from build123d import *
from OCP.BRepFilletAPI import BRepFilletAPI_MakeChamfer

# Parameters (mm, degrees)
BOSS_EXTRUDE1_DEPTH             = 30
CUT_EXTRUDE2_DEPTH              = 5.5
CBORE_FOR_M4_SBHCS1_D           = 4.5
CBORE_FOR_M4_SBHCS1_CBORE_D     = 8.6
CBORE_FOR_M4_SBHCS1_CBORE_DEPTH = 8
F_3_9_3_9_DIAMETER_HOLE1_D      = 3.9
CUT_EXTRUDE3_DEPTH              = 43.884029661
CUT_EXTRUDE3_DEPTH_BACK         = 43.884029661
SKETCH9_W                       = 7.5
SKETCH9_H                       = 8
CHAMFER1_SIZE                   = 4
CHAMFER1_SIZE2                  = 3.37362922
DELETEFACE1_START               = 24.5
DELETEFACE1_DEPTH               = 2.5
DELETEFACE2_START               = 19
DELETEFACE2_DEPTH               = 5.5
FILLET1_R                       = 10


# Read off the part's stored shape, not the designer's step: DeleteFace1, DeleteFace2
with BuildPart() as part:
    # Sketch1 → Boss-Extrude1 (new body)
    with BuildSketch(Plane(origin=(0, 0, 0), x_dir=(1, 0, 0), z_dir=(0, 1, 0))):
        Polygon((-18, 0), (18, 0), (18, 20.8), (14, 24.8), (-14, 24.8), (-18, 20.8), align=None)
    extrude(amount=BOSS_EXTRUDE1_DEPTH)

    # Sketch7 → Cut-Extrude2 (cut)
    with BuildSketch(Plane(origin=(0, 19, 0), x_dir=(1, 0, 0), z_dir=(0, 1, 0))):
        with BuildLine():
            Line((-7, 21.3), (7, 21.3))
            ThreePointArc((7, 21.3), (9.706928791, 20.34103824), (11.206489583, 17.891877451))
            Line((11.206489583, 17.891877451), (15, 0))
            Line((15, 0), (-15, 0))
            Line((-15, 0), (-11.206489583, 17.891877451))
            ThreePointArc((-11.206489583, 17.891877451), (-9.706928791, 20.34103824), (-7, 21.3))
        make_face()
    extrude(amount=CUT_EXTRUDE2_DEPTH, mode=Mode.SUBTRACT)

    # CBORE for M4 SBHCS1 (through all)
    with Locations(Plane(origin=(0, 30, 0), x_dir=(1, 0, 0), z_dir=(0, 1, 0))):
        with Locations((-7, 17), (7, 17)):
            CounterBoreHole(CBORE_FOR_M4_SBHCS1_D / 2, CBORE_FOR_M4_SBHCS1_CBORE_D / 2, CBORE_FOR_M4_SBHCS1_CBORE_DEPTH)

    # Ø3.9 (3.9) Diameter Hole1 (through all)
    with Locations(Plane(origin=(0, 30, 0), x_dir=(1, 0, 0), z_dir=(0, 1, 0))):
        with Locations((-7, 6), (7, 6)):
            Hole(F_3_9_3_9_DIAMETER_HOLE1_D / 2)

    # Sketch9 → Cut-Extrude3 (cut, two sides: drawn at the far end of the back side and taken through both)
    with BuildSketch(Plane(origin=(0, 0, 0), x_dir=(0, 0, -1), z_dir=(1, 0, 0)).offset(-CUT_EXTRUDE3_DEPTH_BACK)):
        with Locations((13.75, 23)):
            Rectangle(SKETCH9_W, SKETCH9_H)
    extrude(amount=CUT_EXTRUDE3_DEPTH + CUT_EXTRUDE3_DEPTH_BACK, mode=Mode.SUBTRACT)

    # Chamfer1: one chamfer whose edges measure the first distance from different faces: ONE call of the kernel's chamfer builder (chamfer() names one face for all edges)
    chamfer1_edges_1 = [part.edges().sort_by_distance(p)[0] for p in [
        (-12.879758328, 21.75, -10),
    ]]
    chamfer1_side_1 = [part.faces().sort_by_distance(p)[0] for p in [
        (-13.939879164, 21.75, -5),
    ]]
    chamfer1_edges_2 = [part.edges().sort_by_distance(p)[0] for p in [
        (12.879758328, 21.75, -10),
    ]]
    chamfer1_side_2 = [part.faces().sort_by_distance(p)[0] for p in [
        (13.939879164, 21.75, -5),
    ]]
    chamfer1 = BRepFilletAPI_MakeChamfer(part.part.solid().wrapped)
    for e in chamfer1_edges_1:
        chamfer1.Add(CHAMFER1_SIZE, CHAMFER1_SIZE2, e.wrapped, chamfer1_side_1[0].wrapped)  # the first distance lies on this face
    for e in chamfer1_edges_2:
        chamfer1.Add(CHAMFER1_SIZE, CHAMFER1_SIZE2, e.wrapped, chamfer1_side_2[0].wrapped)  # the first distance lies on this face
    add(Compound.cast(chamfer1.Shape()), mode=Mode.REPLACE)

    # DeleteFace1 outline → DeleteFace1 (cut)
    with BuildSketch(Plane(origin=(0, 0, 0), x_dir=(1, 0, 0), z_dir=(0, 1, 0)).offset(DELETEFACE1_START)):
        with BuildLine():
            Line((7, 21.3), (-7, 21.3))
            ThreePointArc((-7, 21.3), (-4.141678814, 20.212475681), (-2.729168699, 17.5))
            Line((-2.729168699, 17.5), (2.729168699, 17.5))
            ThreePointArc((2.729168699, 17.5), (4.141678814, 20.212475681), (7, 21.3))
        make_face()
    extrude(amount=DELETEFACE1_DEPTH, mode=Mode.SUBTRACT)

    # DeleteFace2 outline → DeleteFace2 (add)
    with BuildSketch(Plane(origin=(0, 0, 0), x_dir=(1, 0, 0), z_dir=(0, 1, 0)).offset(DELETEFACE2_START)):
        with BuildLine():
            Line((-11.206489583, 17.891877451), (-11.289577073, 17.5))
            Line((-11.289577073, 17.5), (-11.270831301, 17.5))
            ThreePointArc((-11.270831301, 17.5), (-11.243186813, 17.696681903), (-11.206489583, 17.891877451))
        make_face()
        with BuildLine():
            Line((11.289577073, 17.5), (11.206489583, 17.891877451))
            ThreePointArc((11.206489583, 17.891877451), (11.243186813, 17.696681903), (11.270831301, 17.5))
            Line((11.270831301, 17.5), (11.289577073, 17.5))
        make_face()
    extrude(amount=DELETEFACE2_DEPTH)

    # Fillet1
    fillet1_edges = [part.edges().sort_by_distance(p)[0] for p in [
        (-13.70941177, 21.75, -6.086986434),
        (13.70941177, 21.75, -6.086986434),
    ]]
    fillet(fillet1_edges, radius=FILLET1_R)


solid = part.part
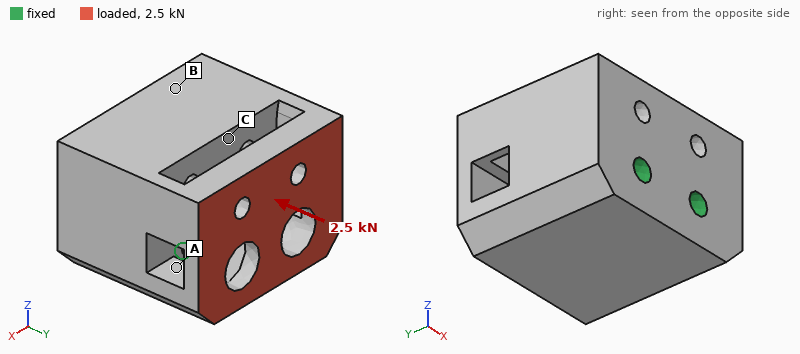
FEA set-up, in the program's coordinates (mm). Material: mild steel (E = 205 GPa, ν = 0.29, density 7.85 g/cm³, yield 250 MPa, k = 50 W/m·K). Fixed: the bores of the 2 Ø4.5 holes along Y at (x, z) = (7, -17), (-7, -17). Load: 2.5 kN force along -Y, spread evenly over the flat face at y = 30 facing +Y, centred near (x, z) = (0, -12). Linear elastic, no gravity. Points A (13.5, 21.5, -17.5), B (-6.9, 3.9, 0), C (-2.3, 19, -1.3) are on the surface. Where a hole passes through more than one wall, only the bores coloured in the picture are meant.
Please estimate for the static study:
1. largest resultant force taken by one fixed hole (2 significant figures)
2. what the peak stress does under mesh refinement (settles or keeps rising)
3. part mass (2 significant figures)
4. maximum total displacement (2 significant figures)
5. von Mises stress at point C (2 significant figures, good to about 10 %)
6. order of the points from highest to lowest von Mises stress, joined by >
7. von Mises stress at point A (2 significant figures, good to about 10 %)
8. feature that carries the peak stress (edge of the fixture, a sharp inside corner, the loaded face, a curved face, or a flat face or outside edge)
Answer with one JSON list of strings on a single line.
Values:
["1.3 kN", "keeps rising", "160 g", "13 µm", "10 MPa", "A > C > B", "21 MPa", "a sharp inside corner"]
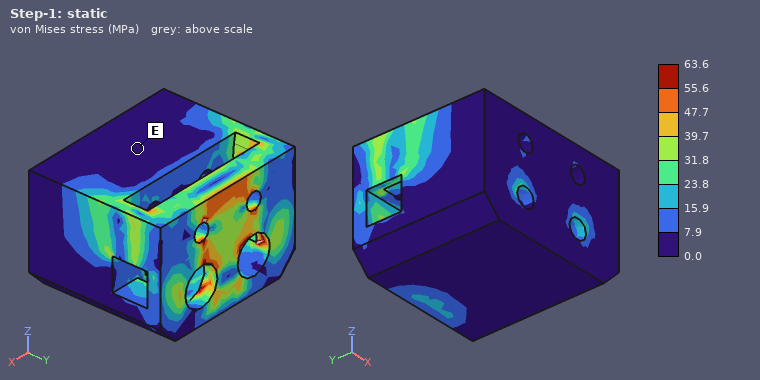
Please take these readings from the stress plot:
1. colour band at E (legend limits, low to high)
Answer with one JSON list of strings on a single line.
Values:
["0.0 to 7.9 MPa"]
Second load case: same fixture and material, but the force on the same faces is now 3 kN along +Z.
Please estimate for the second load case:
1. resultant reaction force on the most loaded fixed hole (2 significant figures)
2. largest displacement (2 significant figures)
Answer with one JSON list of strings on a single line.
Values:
["1.5 kN", "17 µm"]
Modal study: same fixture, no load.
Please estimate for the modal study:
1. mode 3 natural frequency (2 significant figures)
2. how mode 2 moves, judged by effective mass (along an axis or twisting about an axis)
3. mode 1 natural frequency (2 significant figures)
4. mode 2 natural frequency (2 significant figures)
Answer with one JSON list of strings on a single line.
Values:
["18 kHz", "along X", "14 kHz", "15 kHz"]
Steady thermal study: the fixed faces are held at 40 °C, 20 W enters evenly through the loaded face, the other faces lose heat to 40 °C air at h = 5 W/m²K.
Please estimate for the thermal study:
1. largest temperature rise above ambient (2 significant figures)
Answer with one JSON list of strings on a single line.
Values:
["41 K"]
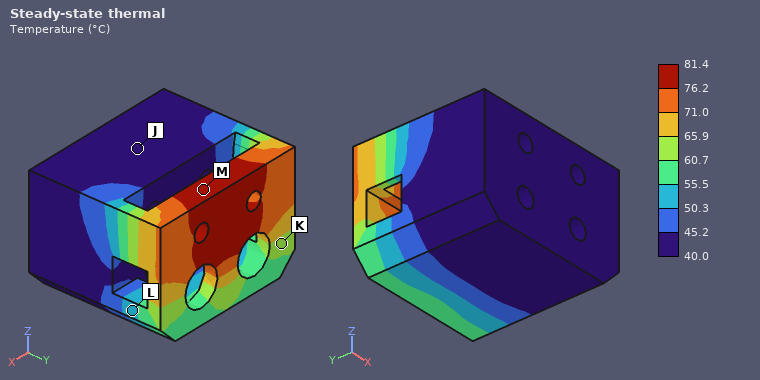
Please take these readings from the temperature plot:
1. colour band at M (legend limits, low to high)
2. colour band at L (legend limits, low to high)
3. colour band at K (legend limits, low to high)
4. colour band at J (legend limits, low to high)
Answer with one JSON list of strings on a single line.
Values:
["76.2 to 81.4 °C", "50.3 to 55.5 °C", "60.7 to 65.9 °C", "40.0 to 45.2 °C"]
